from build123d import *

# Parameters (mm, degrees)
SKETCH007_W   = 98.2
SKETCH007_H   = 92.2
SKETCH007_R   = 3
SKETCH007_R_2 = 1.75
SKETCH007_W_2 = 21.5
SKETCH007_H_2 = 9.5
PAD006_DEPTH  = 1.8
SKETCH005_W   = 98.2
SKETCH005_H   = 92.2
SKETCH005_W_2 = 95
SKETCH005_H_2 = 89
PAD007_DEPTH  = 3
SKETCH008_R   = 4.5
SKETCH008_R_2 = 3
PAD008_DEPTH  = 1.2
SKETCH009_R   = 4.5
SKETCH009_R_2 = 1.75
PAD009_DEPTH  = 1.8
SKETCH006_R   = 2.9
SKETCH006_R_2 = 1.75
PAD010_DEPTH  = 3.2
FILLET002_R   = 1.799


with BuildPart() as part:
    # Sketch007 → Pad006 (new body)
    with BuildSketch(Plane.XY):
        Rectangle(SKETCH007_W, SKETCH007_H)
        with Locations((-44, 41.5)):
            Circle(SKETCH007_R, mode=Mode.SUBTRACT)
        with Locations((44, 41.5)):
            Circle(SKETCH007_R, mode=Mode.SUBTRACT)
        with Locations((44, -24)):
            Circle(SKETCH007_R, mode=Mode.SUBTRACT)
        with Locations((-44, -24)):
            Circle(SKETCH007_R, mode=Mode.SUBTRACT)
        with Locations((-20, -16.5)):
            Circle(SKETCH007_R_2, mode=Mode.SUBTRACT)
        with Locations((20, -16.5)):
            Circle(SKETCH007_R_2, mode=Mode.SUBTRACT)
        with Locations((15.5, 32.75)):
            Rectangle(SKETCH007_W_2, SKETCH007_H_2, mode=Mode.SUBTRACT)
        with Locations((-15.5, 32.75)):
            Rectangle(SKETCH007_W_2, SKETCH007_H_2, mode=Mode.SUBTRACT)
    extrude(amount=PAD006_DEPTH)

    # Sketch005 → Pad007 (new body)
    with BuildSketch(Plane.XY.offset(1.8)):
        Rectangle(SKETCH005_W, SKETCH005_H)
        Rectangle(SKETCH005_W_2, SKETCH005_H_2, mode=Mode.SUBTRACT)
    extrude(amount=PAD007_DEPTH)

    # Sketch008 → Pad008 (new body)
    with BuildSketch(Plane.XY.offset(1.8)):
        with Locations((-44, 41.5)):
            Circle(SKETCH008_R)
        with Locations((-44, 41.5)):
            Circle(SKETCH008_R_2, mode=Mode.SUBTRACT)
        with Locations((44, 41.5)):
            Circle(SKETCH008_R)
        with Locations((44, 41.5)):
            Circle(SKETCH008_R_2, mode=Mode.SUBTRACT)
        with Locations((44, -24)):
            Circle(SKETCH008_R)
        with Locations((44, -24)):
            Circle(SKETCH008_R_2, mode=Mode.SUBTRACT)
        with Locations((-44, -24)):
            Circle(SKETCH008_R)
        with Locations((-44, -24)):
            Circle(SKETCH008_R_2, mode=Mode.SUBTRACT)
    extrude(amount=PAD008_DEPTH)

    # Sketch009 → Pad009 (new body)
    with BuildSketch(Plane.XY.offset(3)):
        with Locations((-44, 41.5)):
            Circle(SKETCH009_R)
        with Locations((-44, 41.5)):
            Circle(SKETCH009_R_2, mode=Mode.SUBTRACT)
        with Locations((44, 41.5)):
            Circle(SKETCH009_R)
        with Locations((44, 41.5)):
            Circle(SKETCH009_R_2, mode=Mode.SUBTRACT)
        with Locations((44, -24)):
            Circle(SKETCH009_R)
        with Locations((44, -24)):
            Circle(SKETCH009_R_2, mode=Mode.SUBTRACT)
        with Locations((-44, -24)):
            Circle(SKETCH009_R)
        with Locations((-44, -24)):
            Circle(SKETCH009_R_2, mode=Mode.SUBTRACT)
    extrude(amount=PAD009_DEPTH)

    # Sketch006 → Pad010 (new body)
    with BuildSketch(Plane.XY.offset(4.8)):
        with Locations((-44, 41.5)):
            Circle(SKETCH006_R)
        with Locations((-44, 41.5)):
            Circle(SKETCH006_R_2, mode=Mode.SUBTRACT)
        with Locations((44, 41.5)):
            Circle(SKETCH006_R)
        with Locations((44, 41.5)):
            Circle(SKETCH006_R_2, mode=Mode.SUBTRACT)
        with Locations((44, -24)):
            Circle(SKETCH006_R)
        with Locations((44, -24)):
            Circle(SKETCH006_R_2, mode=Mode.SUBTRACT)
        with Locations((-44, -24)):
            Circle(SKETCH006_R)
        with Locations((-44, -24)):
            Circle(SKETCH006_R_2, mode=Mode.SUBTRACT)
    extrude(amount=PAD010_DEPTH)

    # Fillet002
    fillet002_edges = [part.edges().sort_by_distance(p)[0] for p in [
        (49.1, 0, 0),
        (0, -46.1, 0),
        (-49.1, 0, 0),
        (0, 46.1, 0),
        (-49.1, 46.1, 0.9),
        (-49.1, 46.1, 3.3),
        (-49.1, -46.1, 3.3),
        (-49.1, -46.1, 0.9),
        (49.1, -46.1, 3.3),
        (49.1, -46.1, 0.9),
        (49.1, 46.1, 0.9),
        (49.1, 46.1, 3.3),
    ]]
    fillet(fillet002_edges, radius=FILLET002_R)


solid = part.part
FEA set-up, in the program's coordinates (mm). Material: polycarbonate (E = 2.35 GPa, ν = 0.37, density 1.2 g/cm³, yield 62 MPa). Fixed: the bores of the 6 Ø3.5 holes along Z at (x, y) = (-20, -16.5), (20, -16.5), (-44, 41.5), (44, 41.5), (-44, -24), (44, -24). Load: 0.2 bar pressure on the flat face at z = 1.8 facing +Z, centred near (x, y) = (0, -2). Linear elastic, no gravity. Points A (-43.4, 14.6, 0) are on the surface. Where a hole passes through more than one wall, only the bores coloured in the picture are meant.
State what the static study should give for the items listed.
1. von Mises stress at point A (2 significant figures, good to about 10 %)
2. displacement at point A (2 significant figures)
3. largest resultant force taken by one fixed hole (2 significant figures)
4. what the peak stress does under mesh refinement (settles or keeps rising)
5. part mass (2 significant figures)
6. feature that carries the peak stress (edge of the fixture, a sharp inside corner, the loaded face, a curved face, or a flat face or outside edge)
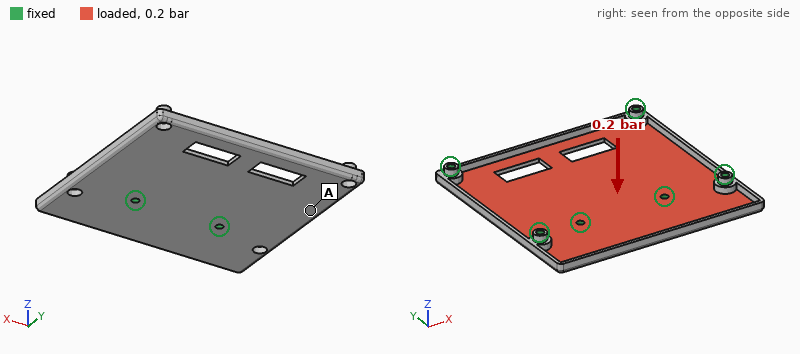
3.0 MPa
0.27 mm
43 N
keeps rising
21 g
edge of the fixture
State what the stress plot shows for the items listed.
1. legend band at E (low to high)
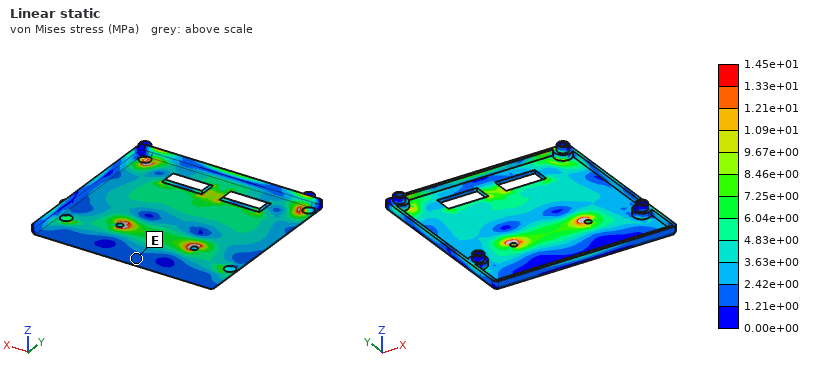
1.21e+00 to 2.42e+00 MPa
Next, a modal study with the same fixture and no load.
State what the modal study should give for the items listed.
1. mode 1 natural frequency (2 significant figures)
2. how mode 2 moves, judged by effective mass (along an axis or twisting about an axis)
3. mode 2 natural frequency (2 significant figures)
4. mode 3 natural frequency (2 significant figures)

500 Hz
along Z
560 Hz
890 Hz
